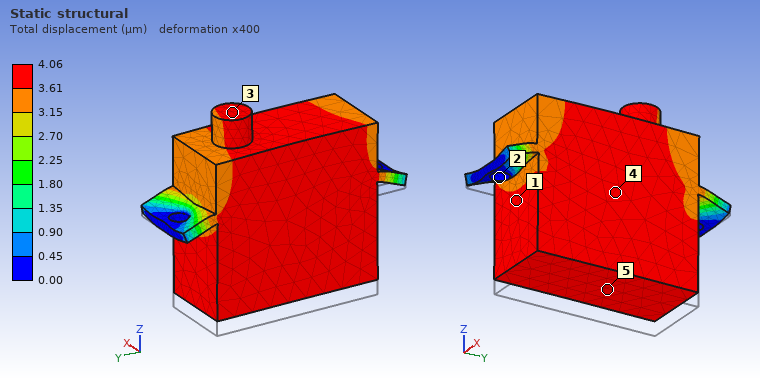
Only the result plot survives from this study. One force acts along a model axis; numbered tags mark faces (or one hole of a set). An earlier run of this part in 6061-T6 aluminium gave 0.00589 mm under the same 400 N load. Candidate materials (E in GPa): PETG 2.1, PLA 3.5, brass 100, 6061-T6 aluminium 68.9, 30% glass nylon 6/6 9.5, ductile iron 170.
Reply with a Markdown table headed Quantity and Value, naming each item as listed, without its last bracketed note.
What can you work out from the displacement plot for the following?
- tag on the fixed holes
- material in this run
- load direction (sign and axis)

| Quantity | Value |
|---|---|
| tag on the fixed holes | 2 |
| material in this run | brass |
| load direction | +Z |
